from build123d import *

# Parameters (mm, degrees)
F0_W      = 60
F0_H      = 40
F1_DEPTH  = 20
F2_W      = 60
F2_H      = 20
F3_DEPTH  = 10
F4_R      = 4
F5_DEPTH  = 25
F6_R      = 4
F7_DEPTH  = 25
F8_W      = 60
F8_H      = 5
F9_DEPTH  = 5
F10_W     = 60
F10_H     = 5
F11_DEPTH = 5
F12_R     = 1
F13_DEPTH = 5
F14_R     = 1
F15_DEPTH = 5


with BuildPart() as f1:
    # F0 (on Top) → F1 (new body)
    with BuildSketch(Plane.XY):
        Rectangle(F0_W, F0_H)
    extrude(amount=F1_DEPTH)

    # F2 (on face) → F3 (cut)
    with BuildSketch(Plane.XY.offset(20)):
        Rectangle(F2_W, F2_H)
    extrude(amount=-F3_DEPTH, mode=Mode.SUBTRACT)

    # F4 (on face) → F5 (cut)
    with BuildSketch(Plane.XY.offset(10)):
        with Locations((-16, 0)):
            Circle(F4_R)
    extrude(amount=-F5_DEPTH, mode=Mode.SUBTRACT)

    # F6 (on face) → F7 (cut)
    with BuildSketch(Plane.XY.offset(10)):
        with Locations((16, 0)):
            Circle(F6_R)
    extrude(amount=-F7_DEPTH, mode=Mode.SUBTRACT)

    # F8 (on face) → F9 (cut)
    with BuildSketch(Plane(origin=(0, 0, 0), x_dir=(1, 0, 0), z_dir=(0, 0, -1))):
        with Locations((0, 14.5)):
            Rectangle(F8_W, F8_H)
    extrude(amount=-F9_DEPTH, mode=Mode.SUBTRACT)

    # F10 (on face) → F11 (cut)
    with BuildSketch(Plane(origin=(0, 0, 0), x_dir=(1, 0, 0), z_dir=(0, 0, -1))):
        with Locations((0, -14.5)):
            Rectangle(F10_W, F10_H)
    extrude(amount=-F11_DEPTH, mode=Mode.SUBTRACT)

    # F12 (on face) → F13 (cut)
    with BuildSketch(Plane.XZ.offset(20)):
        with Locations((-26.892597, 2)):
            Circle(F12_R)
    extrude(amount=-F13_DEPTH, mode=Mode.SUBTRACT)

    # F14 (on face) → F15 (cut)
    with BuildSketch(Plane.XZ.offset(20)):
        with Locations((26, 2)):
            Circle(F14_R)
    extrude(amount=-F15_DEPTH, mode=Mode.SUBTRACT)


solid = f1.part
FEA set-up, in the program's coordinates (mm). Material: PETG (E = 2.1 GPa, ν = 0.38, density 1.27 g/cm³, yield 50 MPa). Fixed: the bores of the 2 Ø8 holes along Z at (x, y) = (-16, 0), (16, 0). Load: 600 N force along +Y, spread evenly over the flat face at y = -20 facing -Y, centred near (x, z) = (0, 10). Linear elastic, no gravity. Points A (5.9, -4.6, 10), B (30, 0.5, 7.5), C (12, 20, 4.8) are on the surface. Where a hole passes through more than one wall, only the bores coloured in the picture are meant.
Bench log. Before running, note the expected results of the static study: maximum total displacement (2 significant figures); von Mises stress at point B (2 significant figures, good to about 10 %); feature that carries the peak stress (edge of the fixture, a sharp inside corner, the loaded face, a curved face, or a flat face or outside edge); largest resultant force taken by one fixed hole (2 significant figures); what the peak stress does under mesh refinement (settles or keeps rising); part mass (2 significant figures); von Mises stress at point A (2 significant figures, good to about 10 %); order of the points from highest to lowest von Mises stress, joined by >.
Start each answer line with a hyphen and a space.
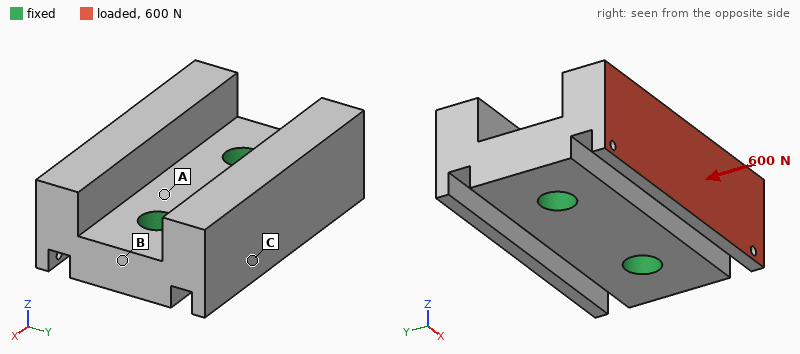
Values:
- 0.11 mm
- 1.3 MPa
- edge of the fixture
- 300 N
- keeps rising
- 41 g
- 2.5 MPa
- A > B > C
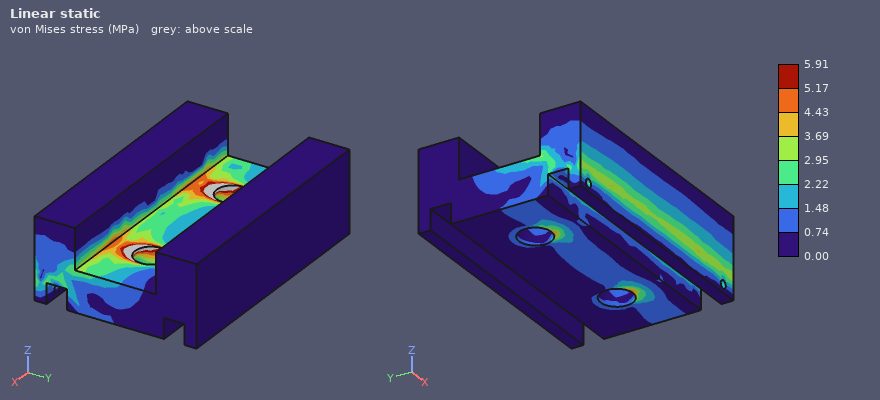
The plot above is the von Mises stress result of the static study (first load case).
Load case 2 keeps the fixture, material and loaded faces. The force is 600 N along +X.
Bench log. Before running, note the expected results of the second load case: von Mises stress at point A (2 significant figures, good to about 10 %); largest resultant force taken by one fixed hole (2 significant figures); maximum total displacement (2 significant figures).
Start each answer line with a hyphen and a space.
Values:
- 2.5 MPa
- 420 N
- 73 µm
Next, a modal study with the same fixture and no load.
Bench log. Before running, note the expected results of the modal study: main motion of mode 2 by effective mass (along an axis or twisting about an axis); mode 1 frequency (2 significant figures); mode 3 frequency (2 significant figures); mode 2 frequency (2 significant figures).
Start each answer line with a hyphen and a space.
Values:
- along Z
- 2400 Hz
- 3300 Hz
- 2800 Hz
